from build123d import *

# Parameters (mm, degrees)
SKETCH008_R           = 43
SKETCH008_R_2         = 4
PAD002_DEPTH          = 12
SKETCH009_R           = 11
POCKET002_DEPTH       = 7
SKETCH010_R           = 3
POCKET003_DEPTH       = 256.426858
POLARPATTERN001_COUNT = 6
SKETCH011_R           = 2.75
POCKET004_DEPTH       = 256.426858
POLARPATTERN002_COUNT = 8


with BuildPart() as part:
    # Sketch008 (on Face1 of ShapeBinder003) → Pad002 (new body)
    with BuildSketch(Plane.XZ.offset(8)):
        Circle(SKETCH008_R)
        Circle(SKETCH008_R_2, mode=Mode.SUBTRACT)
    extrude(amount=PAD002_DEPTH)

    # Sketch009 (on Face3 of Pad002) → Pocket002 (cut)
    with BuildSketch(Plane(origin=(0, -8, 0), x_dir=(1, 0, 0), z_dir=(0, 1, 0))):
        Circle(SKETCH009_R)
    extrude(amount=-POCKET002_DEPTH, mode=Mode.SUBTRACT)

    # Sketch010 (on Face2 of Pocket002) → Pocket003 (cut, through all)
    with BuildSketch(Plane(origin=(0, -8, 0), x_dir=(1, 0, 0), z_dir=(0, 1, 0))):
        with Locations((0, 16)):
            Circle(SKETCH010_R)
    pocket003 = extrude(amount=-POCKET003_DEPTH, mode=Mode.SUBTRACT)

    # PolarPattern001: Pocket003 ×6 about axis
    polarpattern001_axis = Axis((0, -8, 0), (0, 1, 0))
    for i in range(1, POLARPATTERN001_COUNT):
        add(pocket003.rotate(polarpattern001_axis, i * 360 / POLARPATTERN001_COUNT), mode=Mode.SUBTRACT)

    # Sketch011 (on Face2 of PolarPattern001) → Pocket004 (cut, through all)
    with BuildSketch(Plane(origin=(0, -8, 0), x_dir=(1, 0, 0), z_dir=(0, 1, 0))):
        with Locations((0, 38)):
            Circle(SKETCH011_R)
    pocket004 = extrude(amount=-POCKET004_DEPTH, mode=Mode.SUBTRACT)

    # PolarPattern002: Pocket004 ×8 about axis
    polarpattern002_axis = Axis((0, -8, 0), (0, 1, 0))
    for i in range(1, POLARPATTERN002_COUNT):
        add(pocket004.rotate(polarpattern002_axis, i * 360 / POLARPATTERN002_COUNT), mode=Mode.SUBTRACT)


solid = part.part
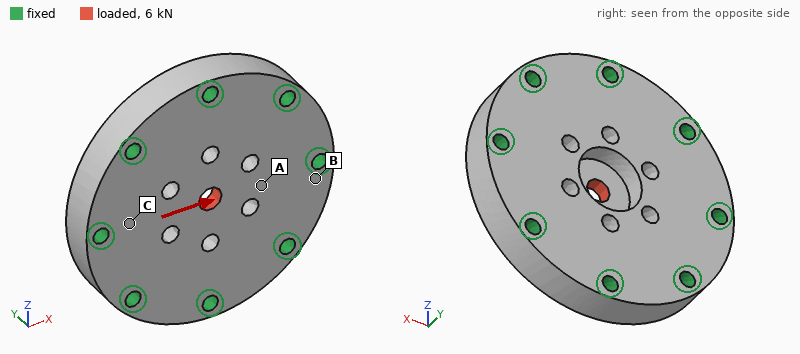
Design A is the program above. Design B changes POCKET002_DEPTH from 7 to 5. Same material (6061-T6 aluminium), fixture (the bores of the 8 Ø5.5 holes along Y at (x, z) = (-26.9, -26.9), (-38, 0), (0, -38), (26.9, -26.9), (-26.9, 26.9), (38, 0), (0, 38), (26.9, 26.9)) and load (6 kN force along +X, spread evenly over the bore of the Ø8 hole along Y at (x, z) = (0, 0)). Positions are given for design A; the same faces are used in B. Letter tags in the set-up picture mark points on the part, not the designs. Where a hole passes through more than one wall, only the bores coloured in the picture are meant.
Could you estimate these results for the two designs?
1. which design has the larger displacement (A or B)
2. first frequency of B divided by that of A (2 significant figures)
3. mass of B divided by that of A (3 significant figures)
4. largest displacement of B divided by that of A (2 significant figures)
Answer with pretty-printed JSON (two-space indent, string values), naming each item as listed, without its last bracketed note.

{
  "which design has the larger displacement": "A",
  "first frequency of B divided by that of A": "0.97",
  "mass of B divided by that of A": "1.01",
  "largest displacement of B divided by that of A": "0.79"
}
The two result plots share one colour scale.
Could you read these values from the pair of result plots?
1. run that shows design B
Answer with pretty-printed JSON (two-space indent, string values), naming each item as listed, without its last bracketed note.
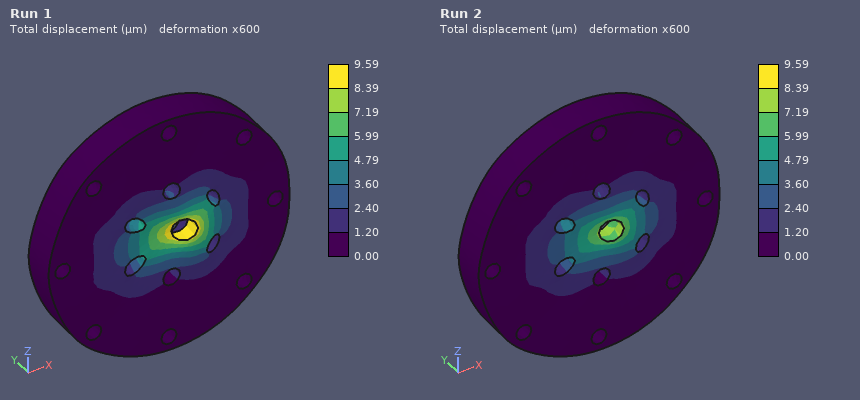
{
  "run that shows design B": "Run 2"
}
